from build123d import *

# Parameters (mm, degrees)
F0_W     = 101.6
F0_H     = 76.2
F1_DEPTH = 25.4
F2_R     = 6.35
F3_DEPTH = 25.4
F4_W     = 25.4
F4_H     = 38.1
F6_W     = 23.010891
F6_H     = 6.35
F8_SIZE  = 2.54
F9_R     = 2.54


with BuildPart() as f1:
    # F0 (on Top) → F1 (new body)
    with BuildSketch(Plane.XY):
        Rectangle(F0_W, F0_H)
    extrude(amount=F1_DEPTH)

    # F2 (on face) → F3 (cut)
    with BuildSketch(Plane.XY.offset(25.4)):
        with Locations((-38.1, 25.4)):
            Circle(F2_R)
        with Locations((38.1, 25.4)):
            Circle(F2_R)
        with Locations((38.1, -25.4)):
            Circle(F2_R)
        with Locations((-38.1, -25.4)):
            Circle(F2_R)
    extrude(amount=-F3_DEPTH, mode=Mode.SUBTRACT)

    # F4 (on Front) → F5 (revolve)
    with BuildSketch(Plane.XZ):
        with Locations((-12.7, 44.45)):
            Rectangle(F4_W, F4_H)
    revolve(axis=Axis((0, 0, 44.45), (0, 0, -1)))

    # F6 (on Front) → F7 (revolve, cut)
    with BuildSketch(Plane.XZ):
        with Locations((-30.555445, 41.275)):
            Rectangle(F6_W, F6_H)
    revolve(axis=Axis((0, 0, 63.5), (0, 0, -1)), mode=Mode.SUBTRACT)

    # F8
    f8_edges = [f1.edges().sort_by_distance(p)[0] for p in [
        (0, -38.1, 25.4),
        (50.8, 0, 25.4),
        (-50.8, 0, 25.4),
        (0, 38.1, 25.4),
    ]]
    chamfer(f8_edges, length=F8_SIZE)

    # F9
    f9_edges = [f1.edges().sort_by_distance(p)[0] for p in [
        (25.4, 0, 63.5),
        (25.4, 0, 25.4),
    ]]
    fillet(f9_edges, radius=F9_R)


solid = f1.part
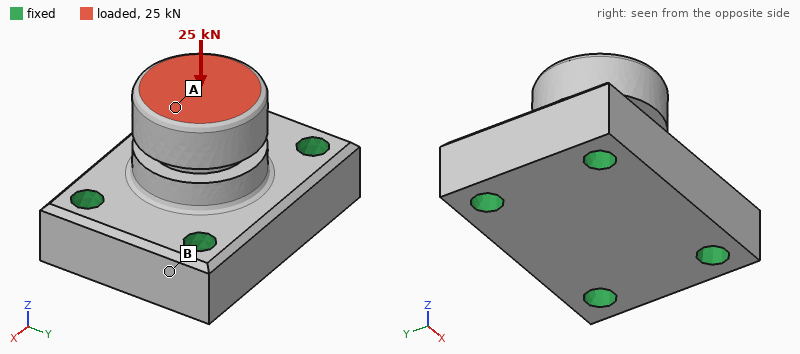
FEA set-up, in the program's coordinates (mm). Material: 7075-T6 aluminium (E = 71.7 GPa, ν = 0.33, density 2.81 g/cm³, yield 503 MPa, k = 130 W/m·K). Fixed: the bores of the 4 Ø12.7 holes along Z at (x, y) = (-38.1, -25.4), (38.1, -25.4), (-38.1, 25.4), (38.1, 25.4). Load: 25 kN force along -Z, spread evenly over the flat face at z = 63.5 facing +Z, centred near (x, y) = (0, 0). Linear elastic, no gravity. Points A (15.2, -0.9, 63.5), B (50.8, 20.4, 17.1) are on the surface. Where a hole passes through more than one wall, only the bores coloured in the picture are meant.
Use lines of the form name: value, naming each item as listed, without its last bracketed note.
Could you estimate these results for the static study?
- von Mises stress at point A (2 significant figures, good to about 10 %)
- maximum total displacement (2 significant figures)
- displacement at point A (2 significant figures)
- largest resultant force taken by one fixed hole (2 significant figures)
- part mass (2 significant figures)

von Mises stress at point A: 15 MPa
maximum total displacement: 19 µm
displacement at point A: 19 µm
largest resultant force taken by one fixed hole: 6.5 kN
part mass: 710 g
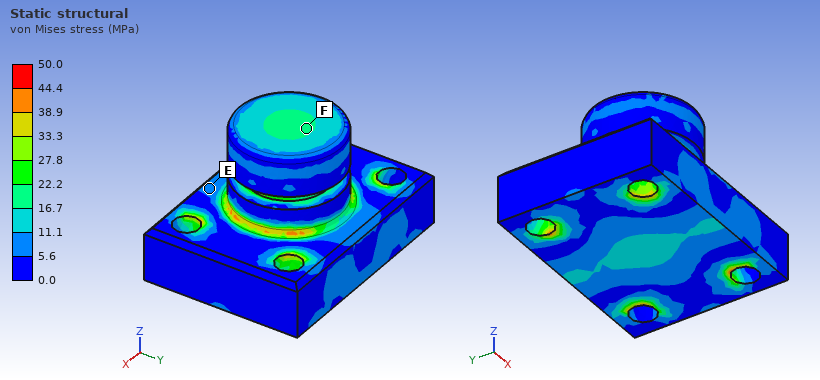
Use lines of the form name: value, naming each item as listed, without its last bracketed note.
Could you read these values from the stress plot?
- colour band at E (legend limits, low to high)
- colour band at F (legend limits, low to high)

colour band at E: 5.6 to 11.1 MPa
colour band at F: 16.7 to 22.2 MPa
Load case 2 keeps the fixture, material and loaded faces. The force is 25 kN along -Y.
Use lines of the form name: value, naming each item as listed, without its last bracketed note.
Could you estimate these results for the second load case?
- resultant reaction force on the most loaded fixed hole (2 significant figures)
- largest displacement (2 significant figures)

resultant reaction force on the most loaded fixed hole: 14 kN
largest displacement: 0.13 mm
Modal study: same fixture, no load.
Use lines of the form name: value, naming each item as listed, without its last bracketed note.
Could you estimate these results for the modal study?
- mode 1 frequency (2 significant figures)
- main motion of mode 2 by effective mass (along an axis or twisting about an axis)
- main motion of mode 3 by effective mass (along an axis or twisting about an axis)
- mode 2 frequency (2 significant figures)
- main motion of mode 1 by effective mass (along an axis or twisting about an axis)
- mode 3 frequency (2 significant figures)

mode 1 frequency: 8000 Hz
main motion of mode 2 by effective mass: along X
main motion of mode 3 by effective mass: along Z
mode 2 frequency: 9400 Hz
main motion of mode 1 by effective mass: along Y
mode 3 frequency: 12 kHz
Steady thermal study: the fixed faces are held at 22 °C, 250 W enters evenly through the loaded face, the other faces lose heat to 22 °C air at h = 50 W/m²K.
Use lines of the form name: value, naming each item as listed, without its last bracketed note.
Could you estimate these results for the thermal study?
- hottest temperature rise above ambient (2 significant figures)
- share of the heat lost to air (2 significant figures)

hottest temperature rise above ambient: 64 K
share of the heat lost to air: 7.9 %
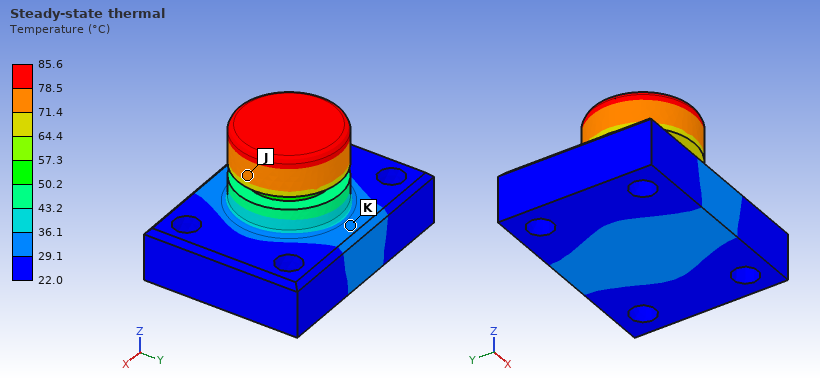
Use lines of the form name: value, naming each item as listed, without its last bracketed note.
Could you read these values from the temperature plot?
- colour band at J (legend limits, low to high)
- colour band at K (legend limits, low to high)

colour band at J: 71.4 to 78.5 °C
colour band at K: 29.1 to 36.1 °C
